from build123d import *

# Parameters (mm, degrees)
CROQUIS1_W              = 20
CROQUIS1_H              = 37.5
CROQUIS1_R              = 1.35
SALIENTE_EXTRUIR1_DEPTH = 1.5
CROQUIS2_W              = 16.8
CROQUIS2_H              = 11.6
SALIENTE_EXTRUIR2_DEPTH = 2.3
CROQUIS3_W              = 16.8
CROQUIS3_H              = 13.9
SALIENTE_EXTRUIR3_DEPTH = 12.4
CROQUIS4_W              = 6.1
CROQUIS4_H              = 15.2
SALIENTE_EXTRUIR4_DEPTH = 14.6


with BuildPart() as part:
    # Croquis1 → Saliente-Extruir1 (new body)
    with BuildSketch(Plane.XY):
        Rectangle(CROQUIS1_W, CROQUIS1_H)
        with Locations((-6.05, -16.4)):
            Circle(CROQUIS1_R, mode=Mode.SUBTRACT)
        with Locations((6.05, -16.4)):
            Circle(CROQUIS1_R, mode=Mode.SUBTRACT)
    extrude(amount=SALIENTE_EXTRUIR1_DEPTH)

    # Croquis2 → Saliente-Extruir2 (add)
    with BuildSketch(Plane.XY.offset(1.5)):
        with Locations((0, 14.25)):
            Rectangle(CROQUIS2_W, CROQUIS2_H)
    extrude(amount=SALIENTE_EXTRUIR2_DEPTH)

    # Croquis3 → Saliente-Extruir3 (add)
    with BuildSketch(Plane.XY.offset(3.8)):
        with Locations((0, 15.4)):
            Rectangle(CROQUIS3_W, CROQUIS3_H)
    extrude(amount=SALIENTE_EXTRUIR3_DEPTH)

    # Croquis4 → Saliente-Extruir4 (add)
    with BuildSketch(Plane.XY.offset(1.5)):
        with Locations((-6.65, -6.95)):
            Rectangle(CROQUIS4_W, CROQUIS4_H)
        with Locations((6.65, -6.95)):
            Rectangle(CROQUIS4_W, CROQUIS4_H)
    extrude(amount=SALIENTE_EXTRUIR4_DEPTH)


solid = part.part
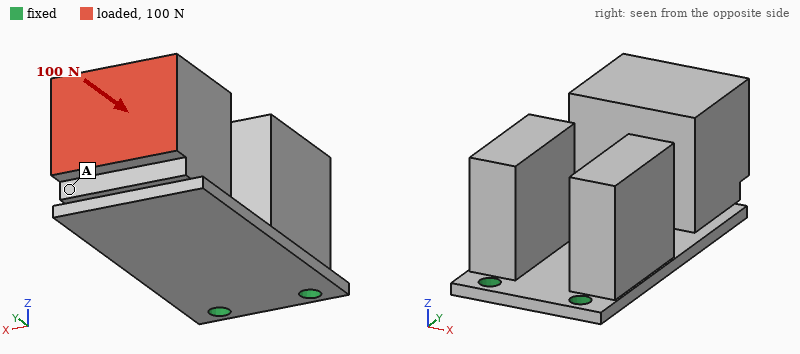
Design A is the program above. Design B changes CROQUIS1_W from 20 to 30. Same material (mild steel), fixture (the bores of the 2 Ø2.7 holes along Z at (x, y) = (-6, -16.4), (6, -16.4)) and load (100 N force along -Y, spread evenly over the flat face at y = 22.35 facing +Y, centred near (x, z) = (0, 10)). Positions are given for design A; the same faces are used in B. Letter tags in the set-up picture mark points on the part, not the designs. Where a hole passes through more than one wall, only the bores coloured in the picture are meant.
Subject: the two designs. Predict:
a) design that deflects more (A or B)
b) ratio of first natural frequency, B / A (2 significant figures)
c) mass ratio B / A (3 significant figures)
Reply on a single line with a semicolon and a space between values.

A; 1.1; 1.08
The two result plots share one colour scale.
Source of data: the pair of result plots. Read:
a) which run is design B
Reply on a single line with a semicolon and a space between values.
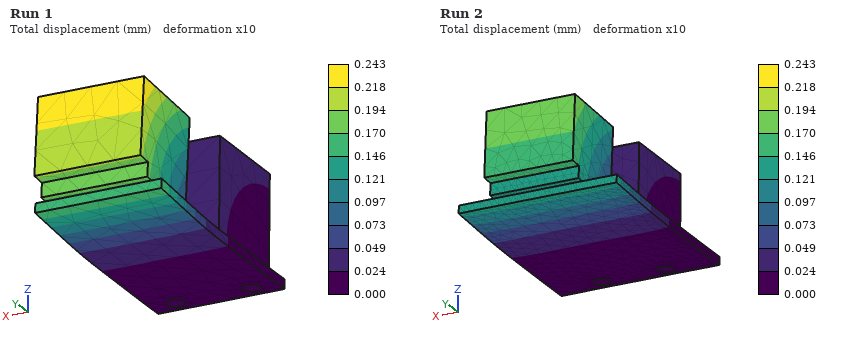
Run 2
